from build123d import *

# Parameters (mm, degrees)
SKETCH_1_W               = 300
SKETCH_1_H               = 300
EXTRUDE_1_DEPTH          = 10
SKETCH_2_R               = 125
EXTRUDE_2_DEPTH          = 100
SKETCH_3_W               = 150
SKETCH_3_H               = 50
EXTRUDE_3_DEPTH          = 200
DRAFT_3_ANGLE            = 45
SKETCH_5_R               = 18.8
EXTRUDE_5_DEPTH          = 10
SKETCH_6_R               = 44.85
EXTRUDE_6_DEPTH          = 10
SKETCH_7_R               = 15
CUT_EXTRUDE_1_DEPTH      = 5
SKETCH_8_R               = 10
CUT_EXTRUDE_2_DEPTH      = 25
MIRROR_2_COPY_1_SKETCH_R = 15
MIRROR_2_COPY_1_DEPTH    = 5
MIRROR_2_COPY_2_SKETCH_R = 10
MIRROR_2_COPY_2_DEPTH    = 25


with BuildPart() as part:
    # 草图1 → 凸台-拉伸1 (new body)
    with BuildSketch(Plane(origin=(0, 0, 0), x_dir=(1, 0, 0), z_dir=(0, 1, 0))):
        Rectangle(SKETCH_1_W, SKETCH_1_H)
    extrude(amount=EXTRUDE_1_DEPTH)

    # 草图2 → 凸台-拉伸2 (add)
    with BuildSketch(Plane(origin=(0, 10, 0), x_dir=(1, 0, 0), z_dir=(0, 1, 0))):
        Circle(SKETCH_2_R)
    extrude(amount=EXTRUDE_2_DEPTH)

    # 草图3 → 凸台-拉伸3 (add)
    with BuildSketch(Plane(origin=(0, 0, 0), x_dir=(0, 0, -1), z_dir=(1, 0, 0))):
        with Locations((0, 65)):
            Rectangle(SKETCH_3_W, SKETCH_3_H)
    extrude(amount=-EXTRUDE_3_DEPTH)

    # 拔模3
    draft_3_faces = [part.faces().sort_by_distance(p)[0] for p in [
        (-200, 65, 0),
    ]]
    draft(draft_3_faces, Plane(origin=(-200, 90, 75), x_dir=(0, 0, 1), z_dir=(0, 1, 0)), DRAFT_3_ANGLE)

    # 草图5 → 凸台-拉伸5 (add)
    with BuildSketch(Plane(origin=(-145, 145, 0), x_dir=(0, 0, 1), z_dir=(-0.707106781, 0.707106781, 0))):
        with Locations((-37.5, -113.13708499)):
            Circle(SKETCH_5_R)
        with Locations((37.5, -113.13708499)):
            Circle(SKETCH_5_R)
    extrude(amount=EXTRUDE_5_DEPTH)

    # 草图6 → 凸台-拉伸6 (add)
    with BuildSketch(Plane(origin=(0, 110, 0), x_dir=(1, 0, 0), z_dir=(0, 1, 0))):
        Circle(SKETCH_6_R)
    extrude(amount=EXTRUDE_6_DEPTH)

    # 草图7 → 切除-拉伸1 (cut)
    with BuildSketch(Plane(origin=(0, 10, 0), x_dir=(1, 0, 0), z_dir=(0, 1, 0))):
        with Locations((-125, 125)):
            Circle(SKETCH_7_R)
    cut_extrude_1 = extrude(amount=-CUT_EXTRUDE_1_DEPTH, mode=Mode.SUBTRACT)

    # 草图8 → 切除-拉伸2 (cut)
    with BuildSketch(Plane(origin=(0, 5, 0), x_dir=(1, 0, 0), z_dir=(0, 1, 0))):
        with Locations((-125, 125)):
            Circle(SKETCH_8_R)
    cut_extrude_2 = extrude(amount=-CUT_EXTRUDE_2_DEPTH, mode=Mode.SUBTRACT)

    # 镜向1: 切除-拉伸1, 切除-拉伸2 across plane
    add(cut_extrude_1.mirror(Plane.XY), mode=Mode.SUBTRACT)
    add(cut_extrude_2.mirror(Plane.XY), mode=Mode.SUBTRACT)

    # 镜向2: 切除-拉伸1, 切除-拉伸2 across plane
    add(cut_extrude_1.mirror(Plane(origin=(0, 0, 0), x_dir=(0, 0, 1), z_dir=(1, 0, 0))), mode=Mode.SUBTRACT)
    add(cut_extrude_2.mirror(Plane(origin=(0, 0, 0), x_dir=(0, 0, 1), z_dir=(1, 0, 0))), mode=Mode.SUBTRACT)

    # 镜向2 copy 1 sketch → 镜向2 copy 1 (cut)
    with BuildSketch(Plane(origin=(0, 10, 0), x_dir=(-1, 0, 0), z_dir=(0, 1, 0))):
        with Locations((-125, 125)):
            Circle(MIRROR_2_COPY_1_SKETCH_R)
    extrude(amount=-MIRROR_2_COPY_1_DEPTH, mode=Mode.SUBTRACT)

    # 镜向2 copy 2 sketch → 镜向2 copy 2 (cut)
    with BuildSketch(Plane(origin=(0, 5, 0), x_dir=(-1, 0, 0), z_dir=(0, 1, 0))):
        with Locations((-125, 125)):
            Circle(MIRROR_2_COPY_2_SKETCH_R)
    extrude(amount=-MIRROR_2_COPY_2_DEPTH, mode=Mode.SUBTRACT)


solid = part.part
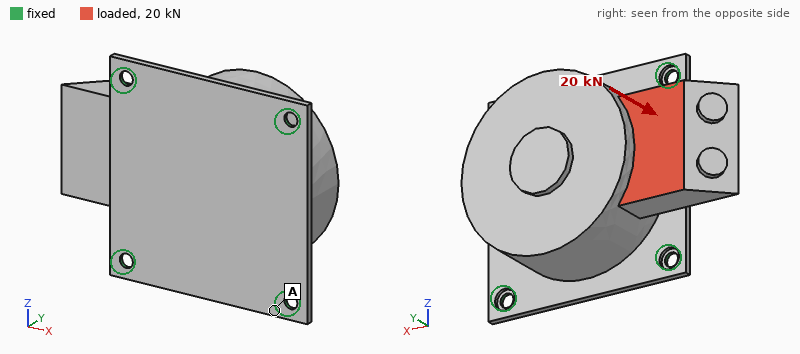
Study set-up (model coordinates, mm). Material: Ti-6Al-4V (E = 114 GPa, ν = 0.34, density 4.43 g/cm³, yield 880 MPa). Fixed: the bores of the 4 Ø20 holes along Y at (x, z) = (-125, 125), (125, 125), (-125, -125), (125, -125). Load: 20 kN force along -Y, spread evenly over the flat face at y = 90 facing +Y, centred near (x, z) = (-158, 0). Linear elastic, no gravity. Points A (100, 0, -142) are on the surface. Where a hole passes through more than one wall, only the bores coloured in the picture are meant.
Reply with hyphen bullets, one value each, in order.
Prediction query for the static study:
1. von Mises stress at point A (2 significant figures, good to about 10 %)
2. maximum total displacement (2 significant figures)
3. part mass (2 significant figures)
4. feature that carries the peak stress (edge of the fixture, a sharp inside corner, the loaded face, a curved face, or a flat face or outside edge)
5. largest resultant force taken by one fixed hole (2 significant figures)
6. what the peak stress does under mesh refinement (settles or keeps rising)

- 19 MPa
- 0.55 mm
- 30 kg
- edge of the fixture
- 17 kN
- keeps rising
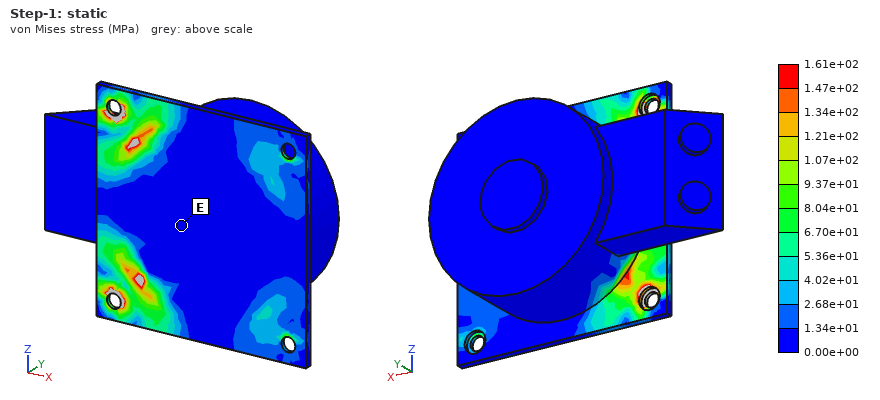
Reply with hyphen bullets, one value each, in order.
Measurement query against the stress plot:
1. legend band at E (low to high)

- 0.00e+00 to 1.34e+01 MPa
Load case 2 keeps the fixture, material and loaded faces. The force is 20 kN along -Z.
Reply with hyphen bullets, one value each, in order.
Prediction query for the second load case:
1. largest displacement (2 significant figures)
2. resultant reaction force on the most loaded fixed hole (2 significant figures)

- 0.13 mm
- 8.9 kN
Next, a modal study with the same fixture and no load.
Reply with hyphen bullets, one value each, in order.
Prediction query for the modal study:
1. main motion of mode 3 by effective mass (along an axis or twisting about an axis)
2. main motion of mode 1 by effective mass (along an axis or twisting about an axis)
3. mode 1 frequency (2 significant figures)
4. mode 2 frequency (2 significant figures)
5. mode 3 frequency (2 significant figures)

- along Z
- along Y
- 360 Hz
- 450 Hz
- 500 Hz
